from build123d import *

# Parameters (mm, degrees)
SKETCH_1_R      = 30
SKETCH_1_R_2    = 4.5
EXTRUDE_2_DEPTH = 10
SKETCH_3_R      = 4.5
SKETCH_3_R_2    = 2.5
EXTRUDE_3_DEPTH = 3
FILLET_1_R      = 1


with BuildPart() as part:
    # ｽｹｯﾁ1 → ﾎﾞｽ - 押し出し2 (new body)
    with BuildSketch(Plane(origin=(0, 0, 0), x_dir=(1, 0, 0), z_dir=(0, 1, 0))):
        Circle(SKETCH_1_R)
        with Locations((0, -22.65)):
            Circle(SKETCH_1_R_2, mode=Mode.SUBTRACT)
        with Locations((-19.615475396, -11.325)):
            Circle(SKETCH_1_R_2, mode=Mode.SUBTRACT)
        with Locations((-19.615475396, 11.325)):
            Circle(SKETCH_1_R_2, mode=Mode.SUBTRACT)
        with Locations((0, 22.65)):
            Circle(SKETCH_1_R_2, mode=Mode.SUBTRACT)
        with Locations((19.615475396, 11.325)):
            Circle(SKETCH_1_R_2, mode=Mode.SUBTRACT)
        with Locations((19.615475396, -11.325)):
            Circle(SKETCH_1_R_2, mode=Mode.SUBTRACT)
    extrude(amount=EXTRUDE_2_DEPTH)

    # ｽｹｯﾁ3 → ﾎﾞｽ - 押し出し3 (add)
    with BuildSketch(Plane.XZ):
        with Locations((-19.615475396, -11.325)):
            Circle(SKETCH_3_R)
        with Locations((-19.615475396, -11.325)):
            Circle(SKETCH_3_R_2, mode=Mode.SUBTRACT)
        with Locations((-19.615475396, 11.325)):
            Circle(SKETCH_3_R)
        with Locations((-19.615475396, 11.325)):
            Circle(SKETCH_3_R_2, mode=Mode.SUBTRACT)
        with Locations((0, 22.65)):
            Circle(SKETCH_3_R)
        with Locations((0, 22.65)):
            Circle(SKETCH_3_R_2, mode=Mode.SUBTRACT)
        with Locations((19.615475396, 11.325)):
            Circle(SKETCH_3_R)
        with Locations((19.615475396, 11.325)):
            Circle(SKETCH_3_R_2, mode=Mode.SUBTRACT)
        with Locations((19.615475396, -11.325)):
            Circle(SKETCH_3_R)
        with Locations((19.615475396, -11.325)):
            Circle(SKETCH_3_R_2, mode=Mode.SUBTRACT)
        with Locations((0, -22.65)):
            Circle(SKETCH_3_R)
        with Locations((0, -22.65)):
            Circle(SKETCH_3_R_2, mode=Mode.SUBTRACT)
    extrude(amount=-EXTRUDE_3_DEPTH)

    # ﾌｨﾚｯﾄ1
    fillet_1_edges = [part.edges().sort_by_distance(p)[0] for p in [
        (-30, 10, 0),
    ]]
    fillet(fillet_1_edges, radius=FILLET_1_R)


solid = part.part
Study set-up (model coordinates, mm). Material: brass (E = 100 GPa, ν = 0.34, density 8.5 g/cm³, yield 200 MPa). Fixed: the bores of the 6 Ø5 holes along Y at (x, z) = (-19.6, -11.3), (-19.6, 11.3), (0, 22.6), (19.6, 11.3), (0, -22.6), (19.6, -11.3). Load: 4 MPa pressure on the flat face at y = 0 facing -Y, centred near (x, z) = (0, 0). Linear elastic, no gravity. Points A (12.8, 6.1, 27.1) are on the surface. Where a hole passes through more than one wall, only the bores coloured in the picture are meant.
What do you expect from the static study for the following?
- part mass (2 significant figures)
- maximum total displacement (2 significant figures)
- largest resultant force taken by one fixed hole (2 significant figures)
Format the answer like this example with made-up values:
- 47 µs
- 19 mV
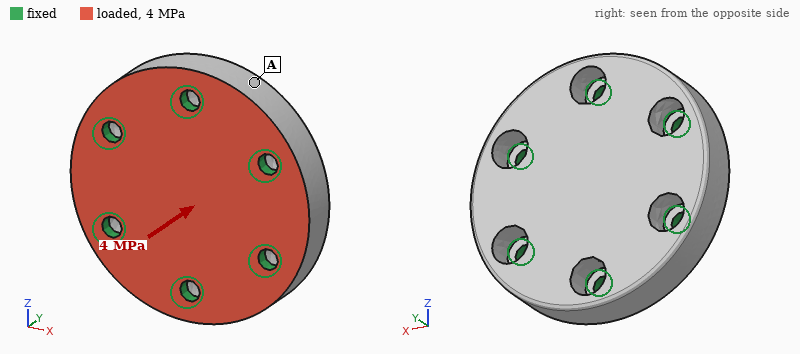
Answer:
- 210 g
- 6.7 µm
- 1.8 kN
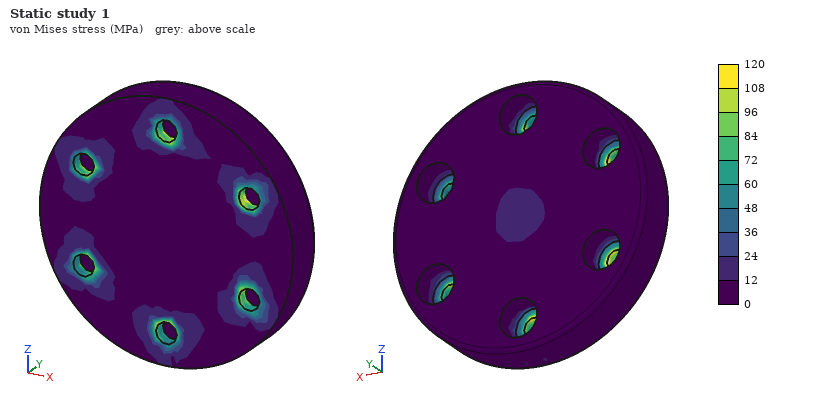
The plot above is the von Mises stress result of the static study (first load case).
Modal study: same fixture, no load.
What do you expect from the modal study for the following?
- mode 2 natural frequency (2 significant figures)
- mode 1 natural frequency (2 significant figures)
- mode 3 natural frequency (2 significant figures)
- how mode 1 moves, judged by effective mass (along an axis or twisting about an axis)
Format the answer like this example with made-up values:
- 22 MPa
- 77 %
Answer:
- 18 kHz
- 16 kHz
- 18 kHz
- along Y
